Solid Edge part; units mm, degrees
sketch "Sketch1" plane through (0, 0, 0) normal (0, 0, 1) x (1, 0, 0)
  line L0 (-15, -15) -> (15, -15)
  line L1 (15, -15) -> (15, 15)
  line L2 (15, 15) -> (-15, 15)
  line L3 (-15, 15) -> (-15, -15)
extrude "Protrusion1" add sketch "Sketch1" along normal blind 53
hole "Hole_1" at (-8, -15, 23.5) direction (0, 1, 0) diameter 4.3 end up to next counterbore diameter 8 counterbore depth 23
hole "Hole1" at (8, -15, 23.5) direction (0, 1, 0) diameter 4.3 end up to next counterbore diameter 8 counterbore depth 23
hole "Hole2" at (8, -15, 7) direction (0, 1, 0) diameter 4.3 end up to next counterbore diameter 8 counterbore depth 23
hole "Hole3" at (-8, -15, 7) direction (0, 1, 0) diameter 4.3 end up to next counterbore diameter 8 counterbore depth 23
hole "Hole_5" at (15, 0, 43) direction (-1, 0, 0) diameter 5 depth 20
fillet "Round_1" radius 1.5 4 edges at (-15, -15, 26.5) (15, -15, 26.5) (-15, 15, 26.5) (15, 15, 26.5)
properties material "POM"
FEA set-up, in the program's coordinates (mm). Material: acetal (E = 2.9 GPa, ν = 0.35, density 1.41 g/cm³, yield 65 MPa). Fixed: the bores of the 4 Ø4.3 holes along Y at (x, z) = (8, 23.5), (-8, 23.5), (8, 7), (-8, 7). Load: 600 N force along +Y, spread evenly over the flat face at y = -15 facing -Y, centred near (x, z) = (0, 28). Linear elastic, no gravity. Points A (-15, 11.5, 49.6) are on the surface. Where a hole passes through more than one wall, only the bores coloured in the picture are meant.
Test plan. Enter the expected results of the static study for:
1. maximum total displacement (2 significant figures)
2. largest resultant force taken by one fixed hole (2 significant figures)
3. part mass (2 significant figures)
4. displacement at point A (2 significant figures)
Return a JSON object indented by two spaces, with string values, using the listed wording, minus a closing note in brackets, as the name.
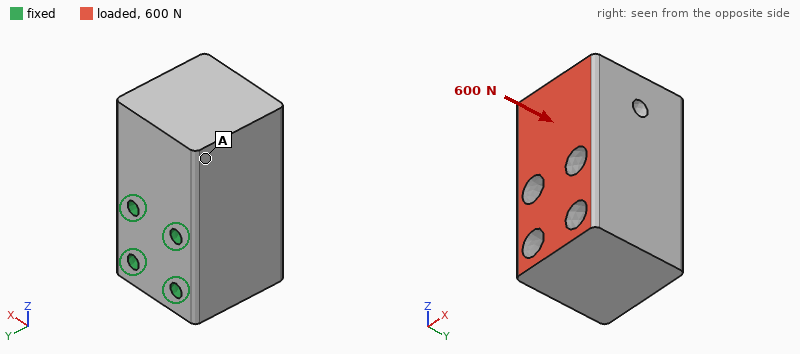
{
  "maximum total displacement": "70 µm",
  "largest resultant force taken by one fixed hole": "340 N",
  "part mass": "59 g",
  "displacement at point A": "52 µm"
}
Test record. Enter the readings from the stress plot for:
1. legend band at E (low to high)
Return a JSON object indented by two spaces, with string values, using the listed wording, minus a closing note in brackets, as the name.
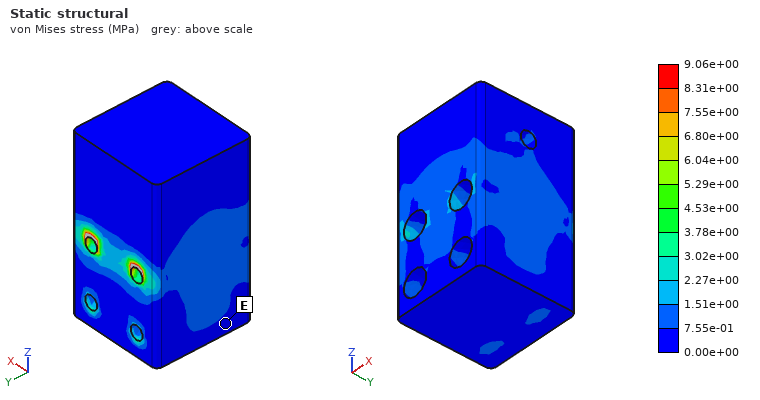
{
  "legend band at E": "0.00e+00 to 7.55e-01 MPa"
}
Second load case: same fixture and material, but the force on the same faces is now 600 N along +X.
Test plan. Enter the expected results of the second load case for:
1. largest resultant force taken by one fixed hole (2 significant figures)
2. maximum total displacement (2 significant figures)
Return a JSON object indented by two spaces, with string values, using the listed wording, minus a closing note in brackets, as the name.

{
  "largest resultant force taken by one fixed hole": "530 N",
  "maximum total displacement": "0.11 mm"
}
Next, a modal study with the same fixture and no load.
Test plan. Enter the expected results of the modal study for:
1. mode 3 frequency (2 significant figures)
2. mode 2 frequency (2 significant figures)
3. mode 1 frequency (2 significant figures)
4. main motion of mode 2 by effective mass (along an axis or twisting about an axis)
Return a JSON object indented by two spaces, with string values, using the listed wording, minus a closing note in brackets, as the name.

{
  "mode 3 frequency": "3900 Hz",
  "mode 2 frequency": "2700 Hz",
  "mode 1 frequency": "2100 Hz",
  "main motion of mode 2 by effective mass": "along X"
}
